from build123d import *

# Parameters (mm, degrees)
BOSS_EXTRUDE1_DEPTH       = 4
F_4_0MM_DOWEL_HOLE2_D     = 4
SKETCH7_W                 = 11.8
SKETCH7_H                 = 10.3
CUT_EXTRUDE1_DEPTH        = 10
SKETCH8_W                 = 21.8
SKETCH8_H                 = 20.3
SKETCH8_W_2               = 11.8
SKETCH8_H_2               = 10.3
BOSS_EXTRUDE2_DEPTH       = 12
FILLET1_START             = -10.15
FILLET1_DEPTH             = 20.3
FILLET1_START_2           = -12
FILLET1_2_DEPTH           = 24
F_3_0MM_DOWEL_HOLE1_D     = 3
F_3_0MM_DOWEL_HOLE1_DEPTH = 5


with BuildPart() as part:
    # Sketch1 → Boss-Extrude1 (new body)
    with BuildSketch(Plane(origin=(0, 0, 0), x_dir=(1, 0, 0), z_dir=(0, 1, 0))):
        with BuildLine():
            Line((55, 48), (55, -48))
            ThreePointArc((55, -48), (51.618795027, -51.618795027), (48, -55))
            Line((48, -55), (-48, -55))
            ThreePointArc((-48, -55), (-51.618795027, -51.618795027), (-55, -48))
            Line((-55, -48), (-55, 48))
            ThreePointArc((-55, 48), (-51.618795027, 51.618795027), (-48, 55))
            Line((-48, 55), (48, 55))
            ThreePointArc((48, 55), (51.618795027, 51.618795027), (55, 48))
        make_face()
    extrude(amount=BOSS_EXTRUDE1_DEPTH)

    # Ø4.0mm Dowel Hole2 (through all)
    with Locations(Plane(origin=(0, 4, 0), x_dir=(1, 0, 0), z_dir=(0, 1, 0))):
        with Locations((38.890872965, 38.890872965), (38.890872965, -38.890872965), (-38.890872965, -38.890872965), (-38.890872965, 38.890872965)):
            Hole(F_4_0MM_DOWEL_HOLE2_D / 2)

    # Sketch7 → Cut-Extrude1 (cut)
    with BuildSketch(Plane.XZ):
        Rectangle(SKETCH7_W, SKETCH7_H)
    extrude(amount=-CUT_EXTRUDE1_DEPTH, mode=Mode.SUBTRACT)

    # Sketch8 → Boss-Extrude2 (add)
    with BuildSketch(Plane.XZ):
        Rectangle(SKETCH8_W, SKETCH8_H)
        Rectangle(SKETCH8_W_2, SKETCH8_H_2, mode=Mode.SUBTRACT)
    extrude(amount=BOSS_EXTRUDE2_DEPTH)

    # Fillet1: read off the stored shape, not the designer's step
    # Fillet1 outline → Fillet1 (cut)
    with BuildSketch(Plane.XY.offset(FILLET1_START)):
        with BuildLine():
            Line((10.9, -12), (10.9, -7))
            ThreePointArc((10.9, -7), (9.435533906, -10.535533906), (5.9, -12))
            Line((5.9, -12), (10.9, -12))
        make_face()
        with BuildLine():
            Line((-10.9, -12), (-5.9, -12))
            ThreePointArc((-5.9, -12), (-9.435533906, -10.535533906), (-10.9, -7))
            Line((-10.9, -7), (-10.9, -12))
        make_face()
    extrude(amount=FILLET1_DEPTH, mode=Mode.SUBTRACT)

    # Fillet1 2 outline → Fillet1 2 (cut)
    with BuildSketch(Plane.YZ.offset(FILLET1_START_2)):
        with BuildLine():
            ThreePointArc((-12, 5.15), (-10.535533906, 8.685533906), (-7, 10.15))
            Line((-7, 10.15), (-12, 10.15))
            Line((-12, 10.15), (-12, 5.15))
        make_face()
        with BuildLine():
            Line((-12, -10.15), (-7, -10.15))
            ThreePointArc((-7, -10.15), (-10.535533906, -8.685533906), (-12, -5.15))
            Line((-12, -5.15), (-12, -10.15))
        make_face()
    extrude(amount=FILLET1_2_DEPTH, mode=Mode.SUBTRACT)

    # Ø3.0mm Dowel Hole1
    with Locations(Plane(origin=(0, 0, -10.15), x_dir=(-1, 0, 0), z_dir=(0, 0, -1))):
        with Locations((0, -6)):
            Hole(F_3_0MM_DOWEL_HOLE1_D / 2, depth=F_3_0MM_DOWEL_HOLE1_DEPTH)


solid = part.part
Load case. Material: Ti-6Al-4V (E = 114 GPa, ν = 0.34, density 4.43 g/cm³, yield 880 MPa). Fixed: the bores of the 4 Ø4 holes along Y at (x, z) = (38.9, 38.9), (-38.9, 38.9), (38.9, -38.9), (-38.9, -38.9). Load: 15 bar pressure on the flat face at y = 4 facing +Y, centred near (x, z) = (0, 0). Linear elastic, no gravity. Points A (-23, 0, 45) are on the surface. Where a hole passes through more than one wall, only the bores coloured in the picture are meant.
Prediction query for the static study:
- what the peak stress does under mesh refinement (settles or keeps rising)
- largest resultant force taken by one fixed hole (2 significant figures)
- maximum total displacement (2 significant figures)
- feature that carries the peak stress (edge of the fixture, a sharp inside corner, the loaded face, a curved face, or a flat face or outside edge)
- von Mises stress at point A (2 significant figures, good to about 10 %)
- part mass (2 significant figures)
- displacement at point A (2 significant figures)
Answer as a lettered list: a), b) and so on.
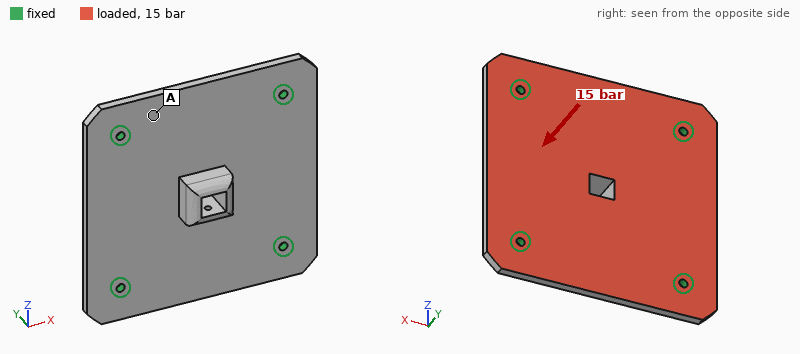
a) keeps rising
b) 4.4 kN
c) 0.48 mm
d) edge of the fixture
e) 71 MPa
f) 220 g
g) 0.13 mm
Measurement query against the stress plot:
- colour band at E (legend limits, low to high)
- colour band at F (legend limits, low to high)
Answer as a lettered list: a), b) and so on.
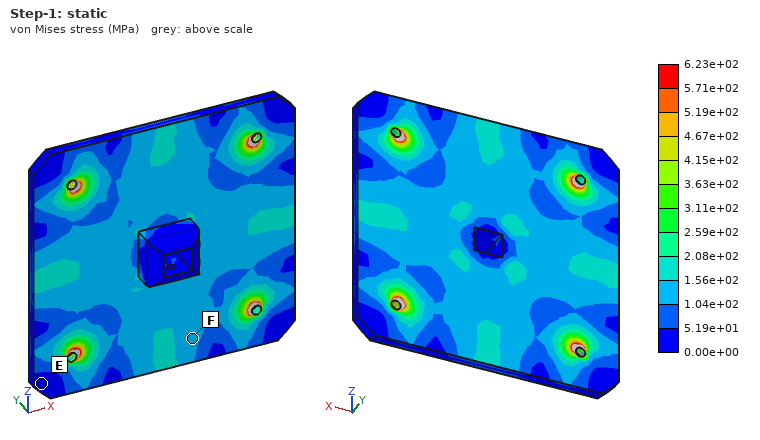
a) 0.00e+00 to 5.19e+01 MPa
b) 1.04e+02 to 1.56e+02 MPa
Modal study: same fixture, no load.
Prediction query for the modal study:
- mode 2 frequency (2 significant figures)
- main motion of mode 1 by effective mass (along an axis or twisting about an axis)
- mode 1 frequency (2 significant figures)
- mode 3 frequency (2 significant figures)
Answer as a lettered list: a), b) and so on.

a) 3400 Hz
b) along Y
c) 2200 Hz
d) 3400 Hz
